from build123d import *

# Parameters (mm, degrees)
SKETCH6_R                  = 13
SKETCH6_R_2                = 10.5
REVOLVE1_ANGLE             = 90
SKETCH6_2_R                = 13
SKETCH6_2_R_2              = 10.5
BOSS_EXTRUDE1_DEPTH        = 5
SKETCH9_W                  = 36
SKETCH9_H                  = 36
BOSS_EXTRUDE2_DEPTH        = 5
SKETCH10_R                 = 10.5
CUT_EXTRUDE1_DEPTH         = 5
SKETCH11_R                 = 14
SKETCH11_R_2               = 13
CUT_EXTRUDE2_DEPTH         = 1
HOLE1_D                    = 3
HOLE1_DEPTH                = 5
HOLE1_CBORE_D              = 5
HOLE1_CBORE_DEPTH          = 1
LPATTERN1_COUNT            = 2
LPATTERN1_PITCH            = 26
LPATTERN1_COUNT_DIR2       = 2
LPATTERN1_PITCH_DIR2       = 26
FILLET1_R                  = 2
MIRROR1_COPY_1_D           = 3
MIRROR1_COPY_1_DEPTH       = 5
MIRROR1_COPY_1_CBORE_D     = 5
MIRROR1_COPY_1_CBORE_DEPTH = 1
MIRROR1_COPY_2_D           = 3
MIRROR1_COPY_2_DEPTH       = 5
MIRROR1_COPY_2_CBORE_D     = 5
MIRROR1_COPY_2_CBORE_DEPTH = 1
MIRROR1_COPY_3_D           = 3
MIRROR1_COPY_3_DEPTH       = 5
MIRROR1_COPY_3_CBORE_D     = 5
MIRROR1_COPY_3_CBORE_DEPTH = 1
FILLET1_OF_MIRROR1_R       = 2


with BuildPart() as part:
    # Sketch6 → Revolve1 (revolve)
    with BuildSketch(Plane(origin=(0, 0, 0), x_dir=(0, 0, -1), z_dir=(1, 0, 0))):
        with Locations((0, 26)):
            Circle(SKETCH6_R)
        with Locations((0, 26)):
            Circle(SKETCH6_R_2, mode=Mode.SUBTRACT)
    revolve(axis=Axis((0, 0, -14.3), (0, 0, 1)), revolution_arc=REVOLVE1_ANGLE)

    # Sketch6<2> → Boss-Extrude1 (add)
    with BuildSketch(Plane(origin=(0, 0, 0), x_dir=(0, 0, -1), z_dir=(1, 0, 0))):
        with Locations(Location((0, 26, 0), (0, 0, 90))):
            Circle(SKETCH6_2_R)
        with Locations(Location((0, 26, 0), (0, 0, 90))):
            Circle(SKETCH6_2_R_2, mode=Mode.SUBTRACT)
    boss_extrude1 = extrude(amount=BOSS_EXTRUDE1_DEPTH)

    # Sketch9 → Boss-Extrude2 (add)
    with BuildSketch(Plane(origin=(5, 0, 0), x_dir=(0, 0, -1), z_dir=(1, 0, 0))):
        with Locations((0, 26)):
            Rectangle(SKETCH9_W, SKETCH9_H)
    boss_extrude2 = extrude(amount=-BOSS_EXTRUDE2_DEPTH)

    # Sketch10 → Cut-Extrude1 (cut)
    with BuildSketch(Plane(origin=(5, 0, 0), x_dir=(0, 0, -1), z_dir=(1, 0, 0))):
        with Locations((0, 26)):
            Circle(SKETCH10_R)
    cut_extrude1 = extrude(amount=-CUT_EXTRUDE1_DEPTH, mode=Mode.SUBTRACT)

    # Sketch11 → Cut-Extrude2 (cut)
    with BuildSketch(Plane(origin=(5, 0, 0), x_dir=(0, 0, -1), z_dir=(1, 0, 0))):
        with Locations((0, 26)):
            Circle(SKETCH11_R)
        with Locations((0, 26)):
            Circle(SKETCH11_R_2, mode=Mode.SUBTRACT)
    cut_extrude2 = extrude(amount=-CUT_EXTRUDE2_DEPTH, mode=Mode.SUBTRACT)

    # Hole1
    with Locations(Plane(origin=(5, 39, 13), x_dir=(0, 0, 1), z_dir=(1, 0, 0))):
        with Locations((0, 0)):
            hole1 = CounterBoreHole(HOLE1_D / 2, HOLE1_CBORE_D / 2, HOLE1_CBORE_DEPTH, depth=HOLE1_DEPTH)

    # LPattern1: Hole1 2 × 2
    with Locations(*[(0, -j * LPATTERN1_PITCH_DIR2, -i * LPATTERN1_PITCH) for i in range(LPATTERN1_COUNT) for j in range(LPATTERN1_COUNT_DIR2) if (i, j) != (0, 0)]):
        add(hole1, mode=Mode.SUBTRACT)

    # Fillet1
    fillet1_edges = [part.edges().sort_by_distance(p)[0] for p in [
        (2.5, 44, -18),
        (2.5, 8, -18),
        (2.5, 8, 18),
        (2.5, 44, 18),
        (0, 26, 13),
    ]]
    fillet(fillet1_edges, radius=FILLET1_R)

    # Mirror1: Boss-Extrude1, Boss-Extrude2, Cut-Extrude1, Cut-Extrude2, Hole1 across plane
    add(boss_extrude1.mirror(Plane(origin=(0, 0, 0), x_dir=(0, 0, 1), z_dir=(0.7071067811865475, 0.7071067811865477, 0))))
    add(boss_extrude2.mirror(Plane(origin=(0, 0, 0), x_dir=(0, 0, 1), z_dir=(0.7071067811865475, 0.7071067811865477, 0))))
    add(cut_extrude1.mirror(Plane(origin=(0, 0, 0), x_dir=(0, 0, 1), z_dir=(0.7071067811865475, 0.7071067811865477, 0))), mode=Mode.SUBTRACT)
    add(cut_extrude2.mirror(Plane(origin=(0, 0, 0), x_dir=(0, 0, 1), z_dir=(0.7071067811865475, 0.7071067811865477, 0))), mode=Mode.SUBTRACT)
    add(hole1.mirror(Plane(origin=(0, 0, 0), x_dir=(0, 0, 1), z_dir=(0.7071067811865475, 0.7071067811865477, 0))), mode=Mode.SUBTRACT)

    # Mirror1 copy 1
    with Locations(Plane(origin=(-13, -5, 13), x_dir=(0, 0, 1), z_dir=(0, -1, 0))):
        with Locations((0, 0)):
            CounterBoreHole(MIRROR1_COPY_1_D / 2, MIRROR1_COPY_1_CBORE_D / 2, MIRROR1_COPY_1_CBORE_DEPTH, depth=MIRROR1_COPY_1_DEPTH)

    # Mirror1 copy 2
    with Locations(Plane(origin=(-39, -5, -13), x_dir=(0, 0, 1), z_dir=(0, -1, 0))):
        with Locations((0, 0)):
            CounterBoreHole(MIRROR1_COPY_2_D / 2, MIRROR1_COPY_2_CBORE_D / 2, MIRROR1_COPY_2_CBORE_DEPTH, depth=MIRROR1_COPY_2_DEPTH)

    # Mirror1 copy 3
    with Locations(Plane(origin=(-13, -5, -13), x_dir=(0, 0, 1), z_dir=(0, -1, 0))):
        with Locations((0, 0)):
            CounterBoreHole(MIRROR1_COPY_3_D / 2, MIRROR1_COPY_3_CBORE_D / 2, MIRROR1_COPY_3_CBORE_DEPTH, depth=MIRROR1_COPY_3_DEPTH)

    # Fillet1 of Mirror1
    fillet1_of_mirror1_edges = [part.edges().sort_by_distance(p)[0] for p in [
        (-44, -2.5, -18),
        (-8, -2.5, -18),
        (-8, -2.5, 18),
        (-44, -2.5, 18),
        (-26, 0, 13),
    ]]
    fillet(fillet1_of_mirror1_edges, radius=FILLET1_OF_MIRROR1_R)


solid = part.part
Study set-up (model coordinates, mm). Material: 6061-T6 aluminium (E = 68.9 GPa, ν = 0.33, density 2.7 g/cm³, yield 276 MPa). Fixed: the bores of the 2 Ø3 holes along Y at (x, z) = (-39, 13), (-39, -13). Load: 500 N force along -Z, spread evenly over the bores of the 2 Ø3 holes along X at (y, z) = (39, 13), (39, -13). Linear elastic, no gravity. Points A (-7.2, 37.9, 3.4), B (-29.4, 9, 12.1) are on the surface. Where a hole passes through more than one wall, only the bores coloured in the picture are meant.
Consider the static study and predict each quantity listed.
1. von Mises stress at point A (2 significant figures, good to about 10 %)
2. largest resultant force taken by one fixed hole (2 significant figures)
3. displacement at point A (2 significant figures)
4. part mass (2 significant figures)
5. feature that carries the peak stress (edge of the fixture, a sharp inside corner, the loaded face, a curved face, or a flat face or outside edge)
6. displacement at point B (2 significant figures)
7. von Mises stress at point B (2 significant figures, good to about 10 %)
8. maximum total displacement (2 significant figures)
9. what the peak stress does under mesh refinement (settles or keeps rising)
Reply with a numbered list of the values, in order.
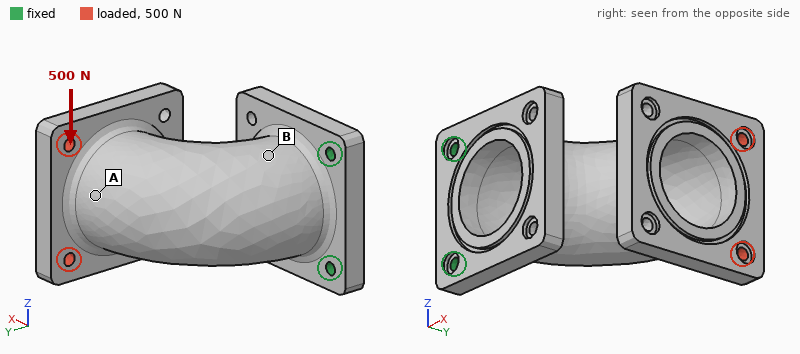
1. 9.4 MPa
2. 1.2 kN
3. 0.085 mm
4. 45 g
5. edge of the fixture
6. 0.024 mm
7. 20 MPa
8. 0.11 mm
9. keeps rising
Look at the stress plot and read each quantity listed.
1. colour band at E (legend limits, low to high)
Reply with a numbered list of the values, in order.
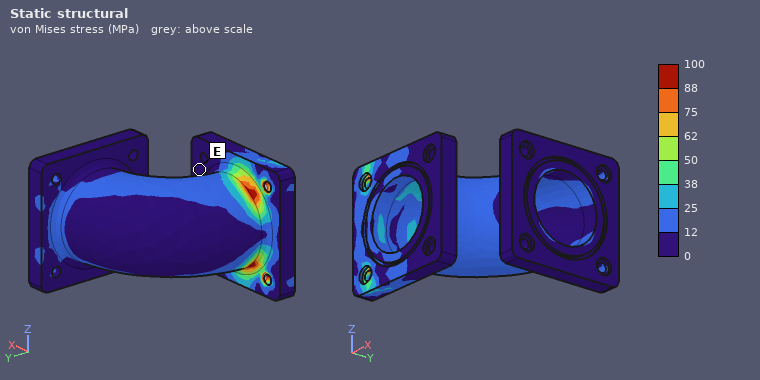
1. 0 to 12 MPa
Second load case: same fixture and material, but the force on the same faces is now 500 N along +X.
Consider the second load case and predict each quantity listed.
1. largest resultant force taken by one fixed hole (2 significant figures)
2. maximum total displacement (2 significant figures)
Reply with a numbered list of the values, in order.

1. 250 N
2. 0.63 mm
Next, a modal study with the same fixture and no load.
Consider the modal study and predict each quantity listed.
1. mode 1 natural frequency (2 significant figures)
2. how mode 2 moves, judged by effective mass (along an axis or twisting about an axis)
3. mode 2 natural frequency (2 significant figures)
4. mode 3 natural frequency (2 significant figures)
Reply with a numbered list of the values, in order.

1. 1000 Hz
2. along Z
3. 3100 Hz
4. 6100 Hz
